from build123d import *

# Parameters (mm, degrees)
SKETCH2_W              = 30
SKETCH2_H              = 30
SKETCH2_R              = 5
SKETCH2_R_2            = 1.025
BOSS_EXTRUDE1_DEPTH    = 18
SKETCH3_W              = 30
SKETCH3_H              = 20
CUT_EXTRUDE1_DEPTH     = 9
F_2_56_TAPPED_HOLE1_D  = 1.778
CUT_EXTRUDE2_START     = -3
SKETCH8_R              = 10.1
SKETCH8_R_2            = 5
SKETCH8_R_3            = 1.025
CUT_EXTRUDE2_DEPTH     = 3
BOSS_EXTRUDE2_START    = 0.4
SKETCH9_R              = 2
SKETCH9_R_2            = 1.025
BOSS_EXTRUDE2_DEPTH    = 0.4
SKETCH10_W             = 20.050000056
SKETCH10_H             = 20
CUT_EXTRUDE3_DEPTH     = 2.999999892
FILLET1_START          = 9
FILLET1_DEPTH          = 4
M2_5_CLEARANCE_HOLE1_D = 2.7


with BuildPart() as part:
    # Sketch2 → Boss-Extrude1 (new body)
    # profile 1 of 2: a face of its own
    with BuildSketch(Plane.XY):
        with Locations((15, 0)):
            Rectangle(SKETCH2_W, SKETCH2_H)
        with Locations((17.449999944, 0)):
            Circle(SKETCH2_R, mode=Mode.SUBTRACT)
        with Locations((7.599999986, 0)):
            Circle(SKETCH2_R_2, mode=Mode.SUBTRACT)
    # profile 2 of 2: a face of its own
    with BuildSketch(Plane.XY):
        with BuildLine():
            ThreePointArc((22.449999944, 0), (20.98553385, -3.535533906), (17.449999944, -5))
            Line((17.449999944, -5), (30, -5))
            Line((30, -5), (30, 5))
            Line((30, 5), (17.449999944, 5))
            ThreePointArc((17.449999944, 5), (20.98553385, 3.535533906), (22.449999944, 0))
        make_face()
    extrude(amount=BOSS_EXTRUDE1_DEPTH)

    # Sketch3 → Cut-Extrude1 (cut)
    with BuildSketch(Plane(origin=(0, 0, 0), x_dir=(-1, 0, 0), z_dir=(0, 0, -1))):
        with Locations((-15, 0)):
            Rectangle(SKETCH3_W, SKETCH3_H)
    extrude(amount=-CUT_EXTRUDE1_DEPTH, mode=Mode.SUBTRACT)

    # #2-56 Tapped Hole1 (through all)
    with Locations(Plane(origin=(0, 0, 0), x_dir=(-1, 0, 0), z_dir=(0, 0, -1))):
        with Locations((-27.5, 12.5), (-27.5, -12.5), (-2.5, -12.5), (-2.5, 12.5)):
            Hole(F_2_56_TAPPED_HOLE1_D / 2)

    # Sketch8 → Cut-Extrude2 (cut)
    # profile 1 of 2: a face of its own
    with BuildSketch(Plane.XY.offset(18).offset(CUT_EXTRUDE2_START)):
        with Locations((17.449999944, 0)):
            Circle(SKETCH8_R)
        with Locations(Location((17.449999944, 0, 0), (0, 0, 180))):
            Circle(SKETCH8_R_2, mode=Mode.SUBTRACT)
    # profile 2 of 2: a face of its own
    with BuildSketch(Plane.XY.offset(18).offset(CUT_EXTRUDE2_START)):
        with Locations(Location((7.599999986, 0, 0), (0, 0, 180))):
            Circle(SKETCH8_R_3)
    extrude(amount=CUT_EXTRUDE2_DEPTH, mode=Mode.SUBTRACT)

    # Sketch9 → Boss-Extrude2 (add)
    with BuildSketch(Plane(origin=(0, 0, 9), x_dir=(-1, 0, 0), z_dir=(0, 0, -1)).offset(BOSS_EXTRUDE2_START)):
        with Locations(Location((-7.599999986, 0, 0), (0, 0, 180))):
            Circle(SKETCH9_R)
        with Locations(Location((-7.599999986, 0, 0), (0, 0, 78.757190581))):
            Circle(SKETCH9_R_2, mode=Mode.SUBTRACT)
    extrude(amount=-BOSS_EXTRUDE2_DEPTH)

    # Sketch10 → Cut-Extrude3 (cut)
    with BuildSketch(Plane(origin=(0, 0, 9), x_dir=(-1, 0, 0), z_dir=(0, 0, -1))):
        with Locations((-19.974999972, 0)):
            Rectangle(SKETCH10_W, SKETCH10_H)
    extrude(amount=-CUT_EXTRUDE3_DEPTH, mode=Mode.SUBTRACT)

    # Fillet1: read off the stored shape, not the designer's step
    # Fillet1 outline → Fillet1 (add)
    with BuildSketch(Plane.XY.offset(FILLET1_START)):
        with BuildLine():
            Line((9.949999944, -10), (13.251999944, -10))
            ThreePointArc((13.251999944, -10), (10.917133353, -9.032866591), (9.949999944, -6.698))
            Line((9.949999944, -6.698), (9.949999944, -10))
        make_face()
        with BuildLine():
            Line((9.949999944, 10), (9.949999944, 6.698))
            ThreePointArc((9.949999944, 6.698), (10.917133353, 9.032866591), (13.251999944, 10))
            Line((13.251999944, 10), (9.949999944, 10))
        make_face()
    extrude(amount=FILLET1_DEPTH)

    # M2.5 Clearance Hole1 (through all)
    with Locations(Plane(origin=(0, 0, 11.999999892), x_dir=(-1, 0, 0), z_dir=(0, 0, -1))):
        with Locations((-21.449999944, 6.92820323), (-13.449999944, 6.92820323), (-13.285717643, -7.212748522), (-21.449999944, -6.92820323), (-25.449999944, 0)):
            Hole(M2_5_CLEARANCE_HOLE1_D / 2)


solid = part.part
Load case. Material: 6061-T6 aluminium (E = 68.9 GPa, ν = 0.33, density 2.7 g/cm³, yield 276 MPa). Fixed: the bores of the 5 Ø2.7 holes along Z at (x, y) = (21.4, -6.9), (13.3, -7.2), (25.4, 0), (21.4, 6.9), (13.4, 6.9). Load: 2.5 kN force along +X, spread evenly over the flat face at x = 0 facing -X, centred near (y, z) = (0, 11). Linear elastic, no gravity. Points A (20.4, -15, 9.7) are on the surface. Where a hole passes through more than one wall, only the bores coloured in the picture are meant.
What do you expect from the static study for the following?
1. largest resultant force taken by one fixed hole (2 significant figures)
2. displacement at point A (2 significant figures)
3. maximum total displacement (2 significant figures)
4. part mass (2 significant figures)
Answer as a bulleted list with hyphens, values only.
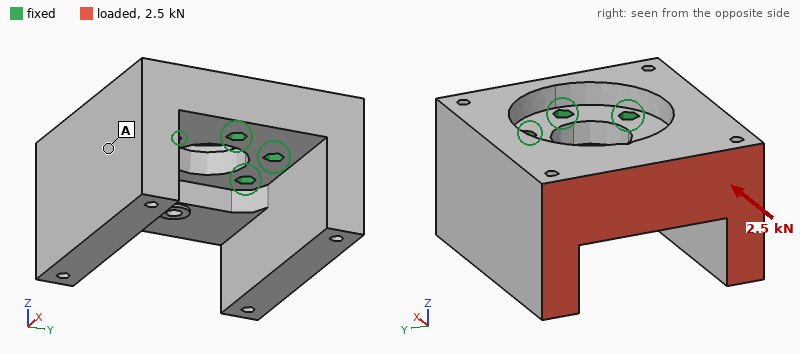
- 970 N
- 3.8 µm
- 13 µm
- 22 g
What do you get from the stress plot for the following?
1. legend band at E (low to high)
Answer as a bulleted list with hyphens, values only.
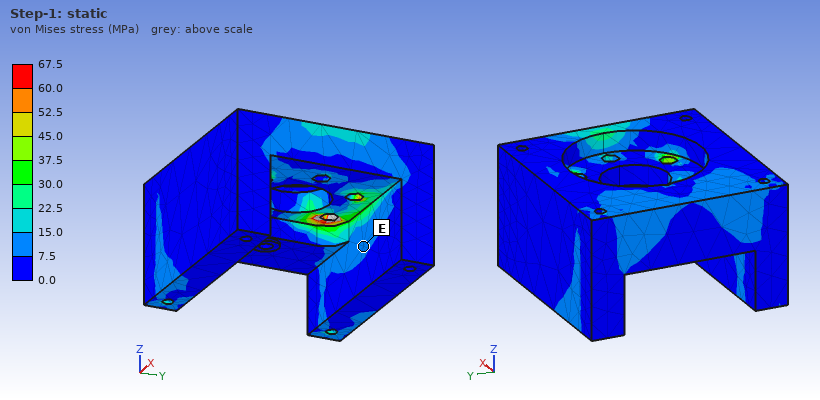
- 7.5 to 15.0 MPa
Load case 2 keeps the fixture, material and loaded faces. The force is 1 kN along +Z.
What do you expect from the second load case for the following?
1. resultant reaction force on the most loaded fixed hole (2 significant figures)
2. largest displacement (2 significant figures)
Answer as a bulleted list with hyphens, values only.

- 940 N
- 34 µm
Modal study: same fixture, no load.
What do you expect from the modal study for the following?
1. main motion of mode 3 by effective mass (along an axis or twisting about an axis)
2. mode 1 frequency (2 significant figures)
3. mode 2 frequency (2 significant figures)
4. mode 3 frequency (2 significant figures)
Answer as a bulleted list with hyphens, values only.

- along Z
- 11 kHz
- 11 kHz
- 13 kHz
